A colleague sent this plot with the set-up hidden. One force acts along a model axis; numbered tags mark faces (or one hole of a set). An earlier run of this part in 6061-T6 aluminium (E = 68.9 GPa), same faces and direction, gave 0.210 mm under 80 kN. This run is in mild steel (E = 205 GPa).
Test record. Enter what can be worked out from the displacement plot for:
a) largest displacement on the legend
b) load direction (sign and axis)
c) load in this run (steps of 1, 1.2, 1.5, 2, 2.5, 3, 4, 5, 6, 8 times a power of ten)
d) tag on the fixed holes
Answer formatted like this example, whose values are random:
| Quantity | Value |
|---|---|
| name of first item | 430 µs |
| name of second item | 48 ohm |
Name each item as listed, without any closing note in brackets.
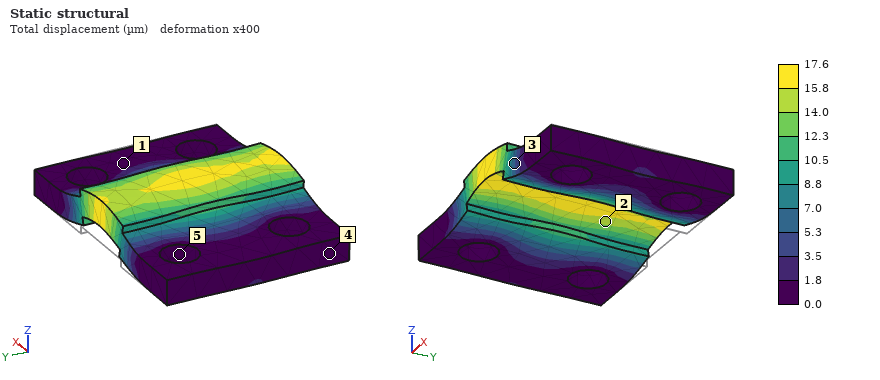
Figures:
| Quantity | Value |
|---|---|
| largest displacement on the legend | 17.6 µm |
| load direction | +Z |
| load in this run | 20 kN |
| tag on the fixed holes | 5 |
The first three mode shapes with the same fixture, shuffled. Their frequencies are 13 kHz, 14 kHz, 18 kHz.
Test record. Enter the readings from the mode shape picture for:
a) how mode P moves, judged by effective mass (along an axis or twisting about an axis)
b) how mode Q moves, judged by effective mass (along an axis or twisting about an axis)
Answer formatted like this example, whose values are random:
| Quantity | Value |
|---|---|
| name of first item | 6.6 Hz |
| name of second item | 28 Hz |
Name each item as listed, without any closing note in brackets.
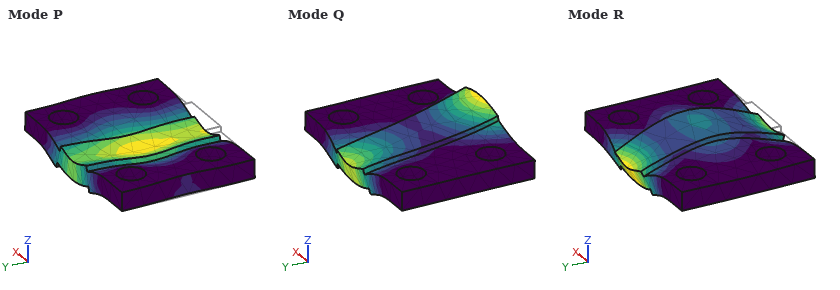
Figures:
| Quantity | Value |
|---|---|
| how mode P moves, judged by effective mass | along Z |
| how mode Q moves, judged by effective mass | twisting about X |
